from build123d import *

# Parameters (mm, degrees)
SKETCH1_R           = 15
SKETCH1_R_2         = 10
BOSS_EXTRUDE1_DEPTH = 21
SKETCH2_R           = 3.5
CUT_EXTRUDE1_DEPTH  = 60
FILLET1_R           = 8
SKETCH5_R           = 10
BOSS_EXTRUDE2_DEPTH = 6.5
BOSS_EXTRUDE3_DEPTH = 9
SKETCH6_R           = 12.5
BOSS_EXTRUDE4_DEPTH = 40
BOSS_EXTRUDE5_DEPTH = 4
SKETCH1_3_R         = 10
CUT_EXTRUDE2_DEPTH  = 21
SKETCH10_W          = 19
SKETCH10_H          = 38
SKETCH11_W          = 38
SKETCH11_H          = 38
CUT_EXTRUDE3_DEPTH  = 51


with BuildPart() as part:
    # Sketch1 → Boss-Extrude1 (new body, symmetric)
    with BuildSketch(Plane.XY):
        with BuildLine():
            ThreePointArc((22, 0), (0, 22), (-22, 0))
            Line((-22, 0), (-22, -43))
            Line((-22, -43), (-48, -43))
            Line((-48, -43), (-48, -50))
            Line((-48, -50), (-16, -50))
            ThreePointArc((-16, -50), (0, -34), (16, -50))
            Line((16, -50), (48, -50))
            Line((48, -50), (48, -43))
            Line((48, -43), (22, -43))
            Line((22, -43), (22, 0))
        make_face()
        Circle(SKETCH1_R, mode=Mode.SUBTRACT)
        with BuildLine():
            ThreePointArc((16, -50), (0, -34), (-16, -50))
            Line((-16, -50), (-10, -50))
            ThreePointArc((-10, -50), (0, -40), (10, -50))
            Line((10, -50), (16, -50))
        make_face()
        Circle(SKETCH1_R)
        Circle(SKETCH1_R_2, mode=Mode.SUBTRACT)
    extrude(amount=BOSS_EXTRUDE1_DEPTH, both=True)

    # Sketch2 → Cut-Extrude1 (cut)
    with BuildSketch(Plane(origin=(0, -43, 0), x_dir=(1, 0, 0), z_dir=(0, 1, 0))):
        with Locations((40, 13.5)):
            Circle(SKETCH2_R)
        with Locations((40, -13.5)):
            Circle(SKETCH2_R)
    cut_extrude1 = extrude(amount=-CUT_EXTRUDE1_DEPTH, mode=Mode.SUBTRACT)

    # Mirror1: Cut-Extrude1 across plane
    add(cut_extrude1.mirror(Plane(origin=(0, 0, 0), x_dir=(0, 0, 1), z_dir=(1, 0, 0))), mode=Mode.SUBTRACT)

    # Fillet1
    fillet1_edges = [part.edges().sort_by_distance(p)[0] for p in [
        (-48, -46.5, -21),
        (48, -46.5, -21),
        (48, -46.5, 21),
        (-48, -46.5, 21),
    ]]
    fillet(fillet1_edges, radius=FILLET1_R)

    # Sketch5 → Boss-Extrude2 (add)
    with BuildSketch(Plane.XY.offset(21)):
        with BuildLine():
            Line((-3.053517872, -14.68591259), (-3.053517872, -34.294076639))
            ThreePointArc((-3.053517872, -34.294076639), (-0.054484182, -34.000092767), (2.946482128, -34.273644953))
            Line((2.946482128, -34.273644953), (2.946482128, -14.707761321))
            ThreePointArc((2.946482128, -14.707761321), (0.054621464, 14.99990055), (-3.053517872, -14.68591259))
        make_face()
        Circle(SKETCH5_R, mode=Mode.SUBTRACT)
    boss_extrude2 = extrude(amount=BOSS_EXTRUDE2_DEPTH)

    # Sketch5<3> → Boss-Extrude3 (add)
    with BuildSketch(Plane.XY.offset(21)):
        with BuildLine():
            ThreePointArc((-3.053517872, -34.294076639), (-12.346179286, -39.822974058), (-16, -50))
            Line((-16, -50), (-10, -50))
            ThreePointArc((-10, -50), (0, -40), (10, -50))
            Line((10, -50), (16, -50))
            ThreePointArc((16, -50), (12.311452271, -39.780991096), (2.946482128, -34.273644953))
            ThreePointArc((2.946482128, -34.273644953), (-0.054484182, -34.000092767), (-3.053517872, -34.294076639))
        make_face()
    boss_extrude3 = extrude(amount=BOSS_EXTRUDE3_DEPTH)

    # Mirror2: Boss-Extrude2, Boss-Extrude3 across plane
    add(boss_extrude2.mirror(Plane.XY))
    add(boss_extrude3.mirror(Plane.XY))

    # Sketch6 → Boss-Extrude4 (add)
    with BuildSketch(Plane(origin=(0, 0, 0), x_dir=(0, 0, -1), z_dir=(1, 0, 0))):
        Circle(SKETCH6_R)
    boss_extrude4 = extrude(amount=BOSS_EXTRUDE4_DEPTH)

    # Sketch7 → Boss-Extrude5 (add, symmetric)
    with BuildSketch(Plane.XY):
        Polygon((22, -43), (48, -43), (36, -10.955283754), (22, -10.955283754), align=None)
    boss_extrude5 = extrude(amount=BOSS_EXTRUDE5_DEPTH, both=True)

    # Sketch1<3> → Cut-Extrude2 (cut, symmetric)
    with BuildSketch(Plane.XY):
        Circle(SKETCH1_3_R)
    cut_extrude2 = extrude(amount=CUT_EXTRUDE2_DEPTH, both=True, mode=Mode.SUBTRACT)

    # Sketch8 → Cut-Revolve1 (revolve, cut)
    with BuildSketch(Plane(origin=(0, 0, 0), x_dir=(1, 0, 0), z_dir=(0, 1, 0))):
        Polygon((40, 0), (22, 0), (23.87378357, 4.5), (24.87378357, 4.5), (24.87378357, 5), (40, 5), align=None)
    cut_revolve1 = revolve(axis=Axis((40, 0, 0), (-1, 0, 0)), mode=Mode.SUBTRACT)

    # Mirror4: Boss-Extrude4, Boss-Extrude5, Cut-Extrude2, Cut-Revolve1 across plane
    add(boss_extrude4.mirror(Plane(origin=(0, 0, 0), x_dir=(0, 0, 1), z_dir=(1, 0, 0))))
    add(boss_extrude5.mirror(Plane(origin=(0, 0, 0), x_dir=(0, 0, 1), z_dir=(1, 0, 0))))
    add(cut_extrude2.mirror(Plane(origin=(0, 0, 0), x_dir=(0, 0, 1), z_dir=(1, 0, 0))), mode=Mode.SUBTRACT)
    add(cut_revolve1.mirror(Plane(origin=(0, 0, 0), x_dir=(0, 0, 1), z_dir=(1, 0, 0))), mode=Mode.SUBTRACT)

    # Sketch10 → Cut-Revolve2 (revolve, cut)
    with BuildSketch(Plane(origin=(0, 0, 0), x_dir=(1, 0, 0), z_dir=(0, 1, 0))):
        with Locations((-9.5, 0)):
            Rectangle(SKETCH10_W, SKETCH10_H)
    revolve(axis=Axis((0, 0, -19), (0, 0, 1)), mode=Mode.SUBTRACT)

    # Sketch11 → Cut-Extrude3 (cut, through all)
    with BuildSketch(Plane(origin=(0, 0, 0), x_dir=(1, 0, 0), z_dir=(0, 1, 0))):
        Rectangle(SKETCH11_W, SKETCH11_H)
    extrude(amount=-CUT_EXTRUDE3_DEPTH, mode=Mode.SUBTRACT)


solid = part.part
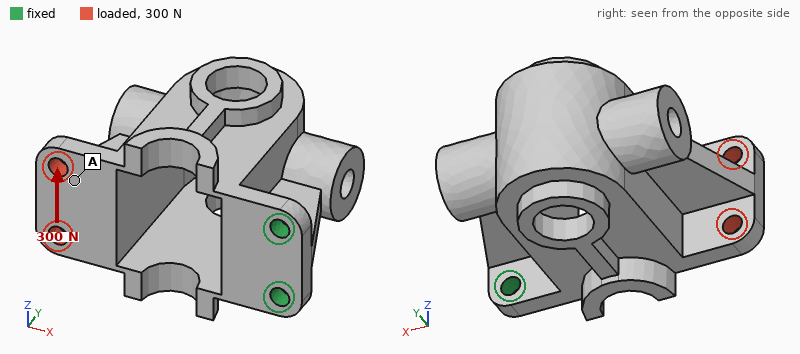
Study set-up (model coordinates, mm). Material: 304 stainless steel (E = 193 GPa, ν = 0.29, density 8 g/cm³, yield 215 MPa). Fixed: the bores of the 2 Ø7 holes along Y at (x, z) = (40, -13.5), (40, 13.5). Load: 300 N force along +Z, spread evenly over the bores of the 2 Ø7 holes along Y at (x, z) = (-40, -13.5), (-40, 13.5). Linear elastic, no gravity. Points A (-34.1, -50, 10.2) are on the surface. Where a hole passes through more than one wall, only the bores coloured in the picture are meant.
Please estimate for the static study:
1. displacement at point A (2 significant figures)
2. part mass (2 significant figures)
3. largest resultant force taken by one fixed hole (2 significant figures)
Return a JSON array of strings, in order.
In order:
["82 µm", "630 g", "790 N"]
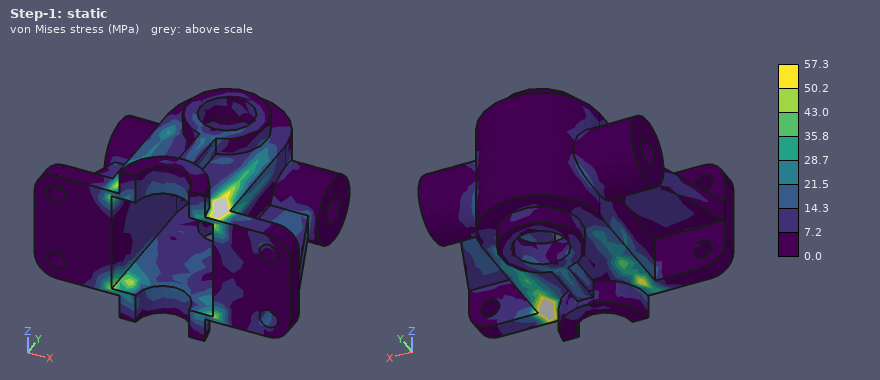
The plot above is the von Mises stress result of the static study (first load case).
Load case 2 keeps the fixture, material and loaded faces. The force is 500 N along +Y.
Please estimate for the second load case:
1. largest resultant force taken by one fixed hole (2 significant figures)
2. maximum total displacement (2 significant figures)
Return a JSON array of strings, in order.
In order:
["290 N", "0.10 mm"]
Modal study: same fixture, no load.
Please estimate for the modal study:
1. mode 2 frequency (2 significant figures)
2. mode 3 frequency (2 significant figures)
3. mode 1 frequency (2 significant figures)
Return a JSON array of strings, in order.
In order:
["690 Hz", "1400 Hz", "670 Hz"]
